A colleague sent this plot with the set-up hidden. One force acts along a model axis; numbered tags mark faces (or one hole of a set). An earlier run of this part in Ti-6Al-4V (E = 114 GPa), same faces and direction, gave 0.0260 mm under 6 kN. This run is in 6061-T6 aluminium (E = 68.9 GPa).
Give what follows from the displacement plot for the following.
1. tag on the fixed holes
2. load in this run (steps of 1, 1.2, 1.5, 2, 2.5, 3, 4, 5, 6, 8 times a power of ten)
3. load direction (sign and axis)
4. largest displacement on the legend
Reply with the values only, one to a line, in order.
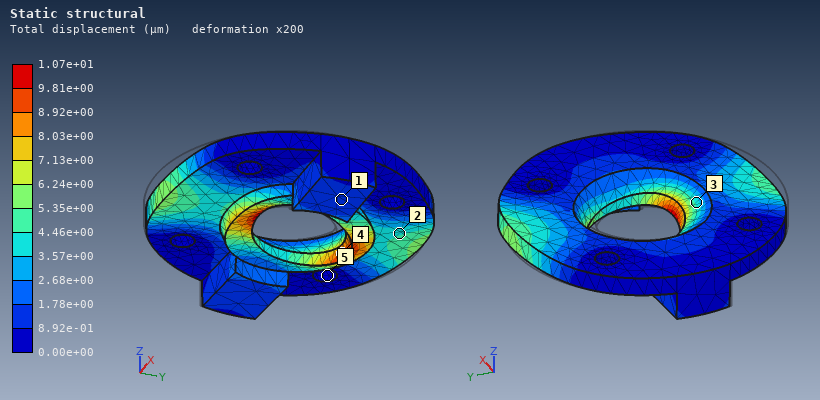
5
1.5 kN
+Y
1.07e+01 µm
